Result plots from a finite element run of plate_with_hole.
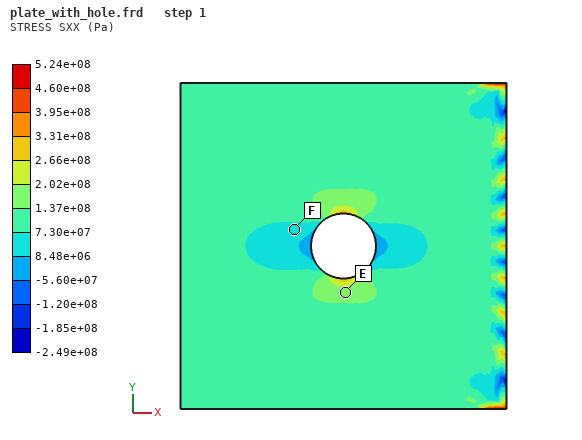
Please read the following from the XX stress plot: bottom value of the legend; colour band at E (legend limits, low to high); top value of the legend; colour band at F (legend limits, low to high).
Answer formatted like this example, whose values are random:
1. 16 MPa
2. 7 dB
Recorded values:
1. -2.49e+08 Pa
2. 1.37e+08 to 2.02e+08 Pa
3. 5.24e+08 Pa
4. 8.48e+06 to 7.30e+07 Pa
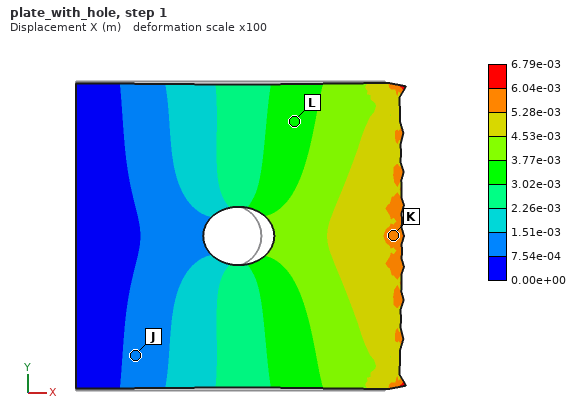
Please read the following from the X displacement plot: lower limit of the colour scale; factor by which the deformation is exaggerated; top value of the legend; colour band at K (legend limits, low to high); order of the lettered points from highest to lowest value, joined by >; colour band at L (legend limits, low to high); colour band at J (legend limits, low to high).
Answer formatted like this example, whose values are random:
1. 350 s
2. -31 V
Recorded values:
1. 0.00e+00 m
2. 100
3. 6.79e-03 m
4. 5.28e-03 to 6.04e-03 m
5. K > L > J
6. 3.02e-03 to 3.77e-03 m
7. 7.54e-04 to 1.51e-03 m
